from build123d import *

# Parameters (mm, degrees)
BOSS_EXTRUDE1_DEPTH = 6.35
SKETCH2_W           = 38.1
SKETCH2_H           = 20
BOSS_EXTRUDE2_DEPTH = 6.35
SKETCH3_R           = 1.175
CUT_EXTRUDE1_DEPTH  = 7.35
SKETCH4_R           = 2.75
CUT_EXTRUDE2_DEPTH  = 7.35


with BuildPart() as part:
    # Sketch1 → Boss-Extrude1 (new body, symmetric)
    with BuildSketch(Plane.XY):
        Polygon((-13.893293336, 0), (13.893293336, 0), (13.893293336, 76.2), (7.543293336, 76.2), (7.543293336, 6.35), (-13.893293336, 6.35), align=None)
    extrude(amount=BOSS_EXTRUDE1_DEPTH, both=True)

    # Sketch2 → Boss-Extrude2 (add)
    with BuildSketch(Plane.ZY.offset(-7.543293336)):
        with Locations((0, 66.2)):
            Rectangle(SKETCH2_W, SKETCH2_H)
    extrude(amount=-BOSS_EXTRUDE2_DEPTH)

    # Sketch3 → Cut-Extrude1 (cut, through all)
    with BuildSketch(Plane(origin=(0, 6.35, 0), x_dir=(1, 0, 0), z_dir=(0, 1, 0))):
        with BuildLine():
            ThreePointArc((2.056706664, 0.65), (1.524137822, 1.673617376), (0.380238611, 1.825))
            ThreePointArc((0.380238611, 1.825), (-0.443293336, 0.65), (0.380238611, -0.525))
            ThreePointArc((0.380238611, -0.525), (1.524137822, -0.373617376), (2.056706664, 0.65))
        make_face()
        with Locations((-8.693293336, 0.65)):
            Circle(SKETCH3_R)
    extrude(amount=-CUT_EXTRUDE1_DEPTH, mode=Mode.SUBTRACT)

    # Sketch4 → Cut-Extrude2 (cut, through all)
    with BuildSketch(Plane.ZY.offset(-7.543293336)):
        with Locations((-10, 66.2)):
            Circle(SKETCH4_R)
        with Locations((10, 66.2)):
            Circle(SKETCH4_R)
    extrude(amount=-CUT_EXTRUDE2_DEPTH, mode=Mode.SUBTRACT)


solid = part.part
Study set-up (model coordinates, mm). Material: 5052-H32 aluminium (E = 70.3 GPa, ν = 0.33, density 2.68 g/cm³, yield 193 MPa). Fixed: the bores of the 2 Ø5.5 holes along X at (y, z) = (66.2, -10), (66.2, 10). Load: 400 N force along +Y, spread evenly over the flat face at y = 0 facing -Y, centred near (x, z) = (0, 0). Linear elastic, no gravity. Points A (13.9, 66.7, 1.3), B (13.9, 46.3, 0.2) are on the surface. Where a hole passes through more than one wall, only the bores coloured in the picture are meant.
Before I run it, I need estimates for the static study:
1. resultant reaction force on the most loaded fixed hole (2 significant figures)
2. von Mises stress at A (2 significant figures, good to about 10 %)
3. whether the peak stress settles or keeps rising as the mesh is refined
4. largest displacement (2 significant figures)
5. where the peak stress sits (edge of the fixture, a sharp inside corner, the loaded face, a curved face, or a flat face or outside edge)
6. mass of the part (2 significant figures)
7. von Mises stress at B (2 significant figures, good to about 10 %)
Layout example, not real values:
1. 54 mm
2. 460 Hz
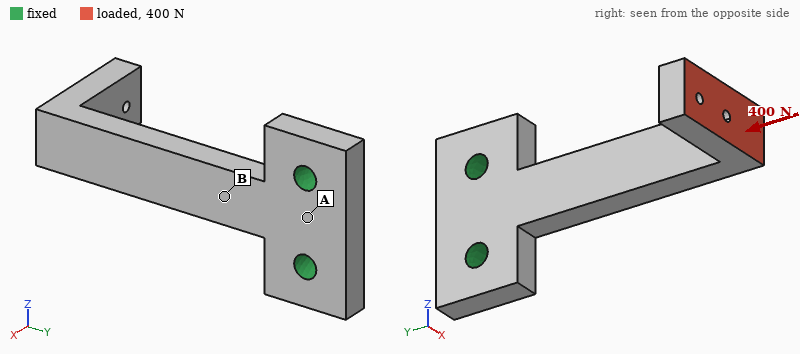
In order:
1. 210 N
2. 8.5 MPa
3. keeps rising
4. 0.56 mm
5. a sharp inside corner
6. 29 g
7. 45 MPa
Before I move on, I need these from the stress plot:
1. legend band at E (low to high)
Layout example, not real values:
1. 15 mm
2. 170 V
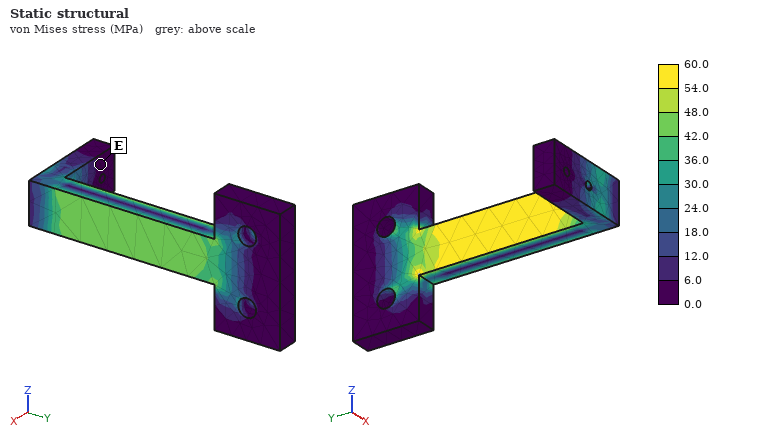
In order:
1. 0.0 to 6.0 MPa
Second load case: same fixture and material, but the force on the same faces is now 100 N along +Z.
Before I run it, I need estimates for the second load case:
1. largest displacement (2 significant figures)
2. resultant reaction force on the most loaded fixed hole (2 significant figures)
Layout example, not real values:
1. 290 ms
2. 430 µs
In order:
1. 0.17 mm
2. 340 N
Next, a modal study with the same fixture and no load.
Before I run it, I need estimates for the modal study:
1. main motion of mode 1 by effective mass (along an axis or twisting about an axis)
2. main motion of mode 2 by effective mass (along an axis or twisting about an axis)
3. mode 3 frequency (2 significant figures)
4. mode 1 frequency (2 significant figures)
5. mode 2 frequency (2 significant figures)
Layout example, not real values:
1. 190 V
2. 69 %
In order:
1. along X
2. along Z
3. 4000 Hz
4. 870 Hz
5. 1700 Hz
